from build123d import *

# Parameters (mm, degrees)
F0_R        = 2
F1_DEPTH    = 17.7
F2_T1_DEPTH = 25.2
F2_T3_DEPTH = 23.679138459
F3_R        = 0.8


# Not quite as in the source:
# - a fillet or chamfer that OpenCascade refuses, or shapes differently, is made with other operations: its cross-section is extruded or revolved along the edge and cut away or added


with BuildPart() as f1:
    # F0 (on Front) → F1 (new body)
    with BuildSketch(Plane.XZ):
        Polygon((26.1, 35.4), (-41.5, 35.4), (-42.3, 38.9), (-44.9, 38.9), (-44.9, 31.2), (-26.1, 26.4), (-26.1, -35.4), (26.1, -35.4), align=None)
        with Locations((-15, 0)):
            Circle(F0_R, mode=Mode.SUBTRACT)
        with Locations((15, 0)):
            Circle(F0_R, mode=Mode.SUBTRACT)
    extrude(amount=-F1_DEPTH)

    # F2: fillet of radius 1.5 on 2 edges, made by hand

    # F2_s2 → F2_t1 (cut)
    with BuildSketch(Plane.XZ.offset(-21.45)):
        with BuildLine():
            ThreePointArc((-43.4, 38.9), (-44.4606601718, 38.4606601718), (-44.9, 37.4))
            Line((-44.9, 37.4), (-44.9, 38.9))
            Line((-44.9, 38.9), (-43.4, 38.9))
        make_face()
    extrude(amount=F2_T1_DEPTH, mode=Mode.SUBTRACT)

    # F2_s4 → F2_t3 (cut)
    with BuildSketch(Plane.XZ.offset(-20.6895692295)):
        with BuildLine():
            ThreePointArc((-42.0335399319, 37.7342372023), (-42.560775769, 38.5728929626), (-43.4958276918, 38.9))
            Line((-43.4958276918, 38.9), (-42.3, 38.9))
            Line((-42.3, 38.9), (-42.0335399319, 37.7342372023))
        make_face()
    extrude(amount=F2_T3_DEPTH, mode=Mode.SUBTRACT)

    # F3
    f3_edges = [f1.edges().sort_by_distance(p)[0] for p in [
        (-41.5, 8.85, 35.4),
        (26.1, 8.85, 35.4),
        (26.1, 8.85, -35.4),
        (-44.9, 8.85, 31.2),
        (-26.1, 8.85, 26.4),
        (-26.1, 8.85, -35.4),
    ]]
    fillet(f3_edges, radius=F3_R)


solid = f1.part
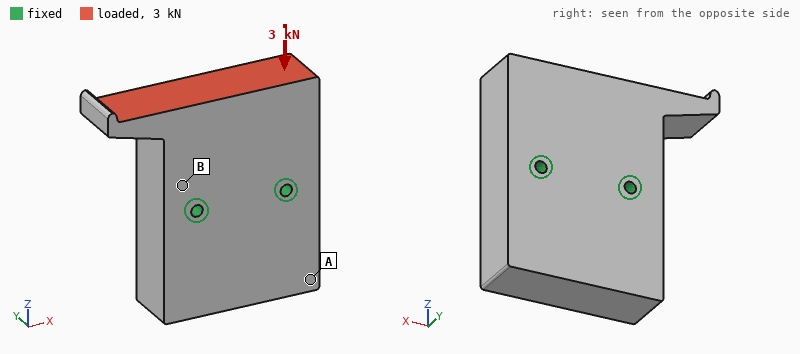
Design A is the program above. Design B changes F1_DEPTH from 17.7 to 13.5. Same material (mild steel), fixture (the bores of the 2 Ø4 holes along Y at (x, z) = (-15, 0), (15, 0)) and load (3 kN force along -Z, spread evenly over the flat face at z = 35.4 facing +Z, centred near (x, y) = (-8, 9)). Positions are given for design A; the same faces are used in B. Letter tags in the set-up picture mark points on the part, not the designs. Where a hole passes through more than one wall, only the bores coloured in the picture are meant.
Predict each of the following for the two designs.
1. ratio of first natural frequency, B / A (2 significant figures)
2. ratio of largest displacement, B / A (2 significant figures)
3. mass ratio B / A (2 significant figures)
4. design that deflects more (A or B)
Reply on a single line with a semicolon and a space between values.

0.82; 1.3; 0.76; B
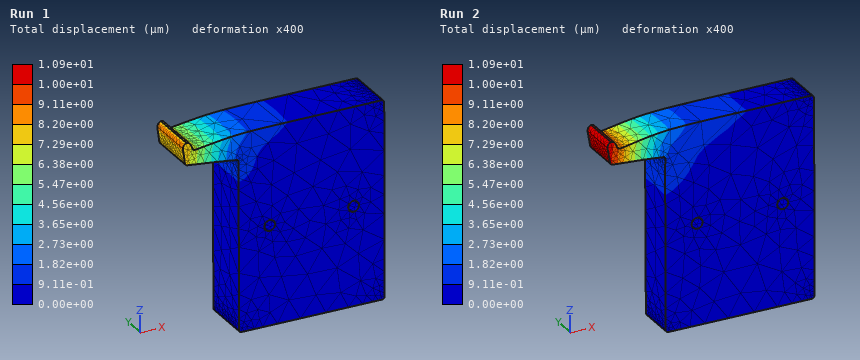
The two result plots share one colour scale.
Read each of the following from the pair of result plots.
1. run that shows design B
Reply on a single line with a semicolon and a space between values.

Run 2
